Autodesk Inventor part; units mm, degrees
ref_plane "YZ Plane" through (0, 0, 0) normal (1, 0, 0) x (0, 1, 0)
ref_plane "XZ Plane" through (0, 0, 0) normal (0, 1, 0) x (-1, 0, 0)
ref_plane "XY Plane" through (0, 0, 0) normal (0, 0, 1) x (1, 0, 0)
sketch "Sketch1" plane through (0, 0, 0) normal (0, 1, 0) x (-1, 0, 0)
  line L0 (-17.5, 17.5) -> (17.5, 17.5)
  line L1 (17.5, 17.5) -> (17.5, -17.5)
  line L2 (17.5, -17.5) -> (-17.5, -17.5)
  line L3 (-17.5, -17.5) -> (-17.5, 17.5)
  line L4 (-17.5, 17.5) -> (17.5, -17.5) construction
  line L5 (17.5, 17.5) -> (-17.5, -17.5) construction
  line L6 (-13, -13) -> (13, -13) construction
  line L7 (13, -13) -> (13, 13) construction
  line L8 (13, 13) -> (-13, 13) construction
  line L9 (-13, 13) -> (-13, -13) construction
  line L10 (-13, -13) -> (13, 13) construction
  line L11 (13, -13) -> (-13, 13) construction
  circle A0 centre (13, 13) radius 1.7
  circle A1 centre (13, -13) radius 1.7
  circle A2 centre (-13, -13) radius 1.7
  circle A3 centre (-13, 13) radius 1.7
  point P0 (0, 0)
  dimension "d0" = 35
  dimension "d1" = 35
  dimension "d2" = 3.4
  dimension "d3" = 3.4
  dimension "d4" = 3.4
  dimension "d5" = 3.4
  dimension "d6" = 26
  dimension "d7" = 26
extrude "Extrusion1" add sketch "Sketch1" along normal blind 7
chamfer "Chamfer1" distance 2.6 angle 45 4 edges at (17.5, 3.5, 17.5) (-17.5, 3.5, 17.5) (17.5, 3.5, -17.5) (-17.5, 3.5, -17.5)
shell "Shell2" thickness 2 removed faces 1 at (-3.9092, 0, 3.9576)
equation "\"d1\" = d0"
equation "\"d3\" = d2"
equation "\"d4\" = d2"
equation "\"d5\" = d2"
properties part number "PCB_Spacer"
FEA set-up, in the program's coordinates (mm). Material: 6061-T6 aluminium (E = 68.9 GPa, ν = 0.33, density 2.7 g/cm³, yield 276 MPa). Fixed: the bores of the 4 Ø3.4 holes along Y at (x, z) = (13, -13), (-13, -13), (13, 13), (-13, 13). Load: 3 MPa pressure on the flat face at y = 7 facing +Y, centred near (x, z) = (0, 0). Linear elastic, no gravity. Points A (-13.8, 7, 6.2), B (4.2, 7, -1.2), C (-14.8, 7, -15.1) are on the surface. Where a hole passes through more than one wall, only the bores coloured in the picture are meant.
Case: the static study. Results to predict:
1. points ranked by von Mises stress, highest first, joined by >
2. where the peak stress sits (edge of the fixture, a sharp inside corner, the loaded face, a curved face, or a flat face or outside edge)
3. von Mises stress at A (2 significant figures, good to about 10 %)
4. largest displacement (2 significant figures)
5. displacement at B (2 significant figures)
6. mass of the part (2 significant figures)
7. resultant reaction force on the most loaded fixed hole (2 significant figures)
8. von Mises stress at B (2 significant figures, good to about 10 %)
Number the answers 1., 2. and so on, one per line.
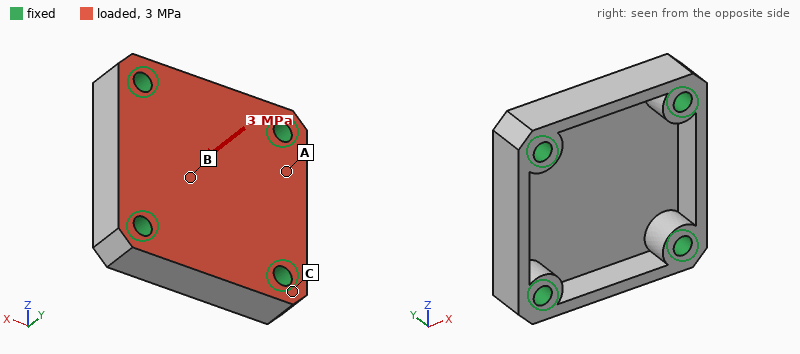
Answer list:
1. B > A > C
2. the loaded face
3. 75 MPa
4. 92 µm
5. 82 µm
6. 11 g
7. 910 N
8. 100 MPa
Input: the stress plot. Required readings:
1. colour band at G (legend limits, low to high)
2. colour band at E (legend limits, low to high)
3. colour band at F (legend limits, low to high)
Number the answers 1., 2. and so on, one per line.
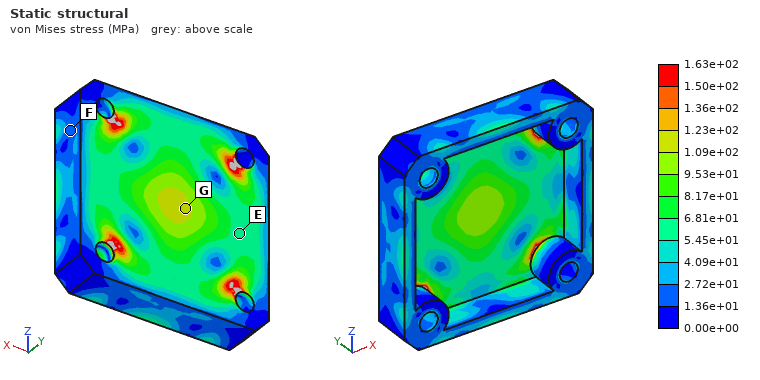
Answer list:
1. 1.09e+02 to 1.23e+02 MPa
2. 5.45e+01 to 6.81e+01 MPa
3. 1.36e+01 to 2.72e+01 MPa
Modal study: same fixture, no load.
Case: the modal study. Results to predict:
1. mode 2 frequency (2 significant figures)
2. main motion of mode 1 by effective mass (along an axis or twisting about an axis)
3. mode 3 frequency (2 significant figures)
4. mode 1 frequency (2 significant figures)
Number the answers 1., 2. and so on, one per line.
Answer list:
1. 29 kHz
2. along Y
3. 29 kHz
4. 15 kHz
